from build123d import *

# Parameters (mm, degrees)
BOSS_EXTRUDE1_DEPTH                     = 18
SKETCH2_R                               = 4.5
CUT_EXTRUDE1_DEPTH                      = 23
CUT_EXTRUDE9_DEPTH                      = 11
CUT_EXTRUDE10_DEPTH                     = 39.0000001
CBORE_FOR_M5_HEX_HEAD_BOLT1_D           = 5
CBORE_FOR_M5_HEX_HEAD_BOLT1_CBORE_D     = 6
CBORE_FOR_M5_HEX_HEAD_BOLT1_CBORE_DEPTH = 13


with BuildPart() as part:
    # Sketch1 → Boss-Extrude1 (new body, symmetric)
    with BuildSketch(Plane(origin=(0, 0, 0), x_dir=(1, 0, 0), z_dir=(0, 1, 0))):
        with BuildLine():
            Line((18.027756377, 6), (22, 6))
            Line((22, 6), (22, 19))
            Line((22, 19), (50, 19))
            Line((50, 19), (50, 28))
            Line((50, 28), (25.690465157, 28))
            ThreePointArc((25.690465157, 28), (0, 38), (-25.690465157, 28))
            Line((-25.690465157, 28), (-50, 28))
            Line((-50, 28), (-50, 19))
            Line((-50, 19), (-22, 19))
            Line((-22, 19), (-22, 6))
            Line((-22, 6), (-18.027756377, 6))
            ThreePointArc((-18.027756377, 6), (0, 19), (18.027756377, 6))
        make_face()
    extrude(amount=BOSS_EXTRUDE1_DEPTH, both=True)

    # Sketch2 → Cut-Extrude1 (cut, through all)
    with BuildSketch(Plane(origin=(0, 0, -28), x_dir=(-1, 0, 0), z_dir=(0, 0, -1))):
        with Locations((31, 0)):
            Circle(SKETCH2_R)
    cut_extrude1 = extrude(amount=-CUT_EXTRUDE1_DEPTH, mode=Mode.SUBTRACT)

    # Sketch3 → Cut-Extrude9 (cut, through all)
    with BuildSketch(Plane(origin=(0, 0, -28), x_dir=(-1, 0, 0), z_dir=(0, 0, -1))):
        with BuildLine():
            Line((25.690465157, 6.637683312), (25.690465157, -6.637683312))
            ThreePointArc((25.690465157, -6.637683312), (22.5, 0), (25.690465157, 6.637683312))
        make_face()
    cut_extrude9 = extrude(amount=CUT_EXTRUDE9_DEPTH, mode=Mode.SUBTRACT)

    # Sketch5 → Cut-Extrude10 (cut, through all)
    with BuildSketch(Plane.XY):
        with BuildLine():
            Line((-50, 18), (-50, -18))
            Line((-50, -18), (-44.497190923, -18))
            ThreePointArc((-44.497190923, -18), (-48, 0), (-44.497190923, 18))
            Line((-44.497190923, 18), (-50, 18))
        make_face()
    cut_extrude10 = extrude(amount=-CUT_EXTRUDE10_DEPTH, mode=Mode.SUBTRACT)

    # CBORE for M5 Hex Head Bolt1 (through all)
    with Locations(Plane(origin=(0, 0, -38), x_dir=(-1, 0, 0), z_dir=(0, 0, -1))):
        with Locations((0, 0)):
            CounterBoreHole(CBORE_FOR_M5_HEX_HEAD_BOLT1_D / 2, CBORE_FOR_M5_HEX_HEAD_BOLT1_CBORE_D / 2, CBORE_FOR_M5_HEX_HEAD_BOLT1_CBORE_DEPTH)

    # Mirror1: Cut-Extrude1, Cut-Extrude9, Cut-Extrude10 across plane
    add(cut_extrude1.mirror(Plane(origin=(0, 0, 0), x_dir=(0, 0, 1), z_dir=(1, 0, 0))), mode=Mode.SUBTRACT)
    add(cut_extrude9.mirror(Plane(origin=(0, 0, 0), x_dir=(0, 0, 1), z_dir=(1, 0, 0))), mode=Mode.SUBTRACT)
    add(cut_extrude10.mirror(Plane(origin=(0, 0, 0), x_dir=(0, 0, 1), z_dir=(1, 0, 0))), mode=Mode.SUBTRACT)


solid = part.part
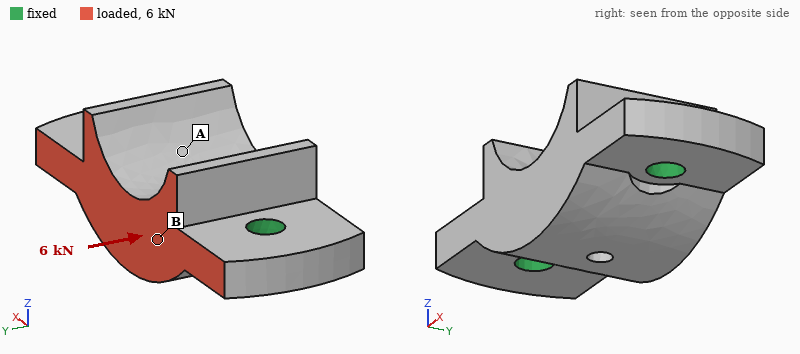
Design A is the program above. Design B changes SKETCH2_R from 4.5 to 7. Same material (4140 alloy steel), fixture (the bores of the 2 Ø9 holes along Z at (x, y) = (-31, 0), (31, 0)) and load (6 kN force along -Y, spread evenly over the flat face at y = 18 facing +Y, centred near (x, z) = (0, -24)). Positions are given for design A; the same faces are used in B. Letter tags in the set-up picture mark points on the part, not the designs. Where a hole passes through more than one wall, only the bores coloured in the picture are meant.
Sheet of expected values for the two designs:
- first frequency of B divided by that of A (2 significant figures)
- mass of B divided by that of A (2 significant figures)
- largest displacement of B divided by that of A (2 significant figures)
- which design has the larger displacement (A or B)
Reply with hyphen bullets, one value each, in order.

- 1.3
- 0.97
- 0.71
- A
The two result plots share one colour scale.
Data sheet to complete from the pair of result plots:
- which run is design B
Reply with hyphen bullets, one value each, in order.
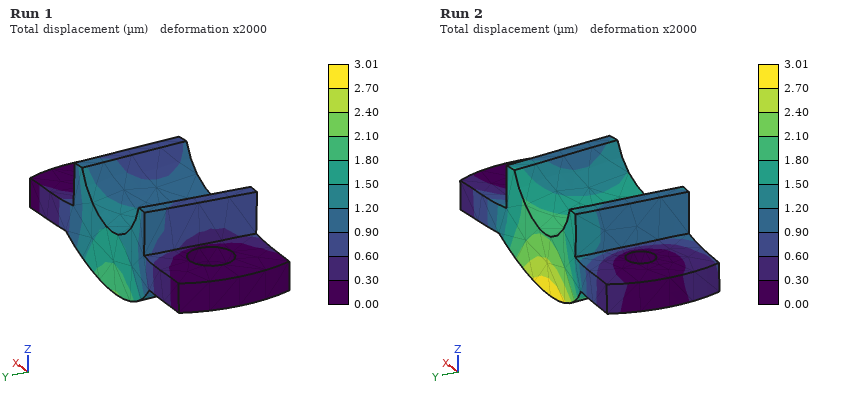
- Run 1
